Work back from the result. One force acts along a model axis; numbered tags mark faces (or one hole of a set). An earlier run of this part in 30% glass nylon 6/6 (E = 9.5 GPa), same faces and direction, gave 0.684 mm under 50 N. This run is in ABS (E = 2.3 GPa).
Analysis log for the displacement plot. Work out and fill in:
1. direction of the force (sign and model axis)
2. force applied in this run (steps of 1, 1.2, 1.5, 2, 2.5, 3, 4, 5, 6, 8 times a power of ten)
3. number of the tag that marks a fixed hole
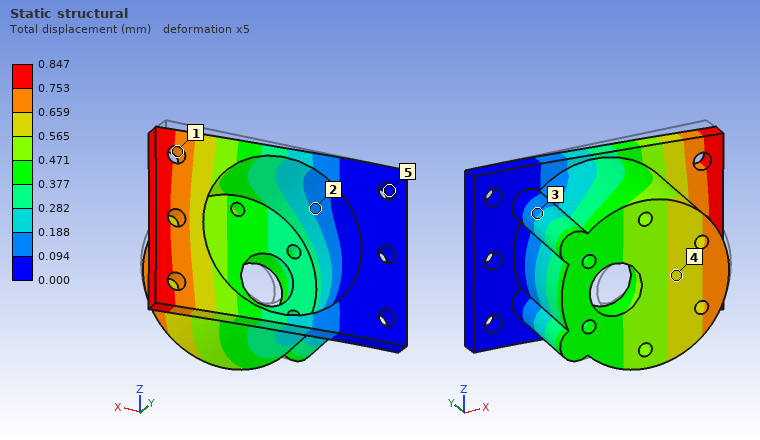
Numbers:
-Y
15 N
5
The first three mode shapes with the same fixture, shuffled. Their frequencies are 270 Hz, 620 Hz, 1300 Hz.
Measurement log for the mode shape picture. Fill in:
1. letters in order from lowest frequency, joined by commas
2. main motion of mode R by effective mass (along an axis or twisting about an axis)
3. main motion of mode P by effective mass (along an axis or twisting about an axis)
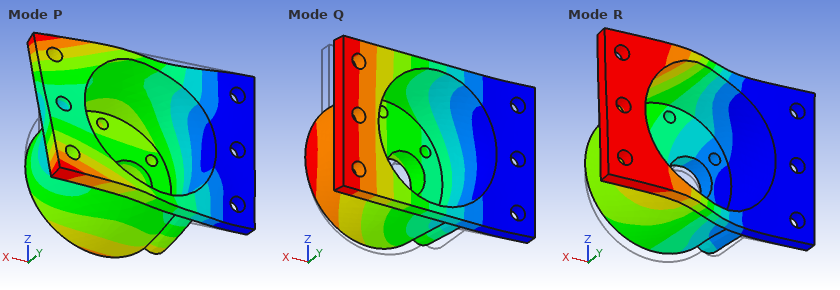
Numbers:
Q, R, P
along Z
along Z
